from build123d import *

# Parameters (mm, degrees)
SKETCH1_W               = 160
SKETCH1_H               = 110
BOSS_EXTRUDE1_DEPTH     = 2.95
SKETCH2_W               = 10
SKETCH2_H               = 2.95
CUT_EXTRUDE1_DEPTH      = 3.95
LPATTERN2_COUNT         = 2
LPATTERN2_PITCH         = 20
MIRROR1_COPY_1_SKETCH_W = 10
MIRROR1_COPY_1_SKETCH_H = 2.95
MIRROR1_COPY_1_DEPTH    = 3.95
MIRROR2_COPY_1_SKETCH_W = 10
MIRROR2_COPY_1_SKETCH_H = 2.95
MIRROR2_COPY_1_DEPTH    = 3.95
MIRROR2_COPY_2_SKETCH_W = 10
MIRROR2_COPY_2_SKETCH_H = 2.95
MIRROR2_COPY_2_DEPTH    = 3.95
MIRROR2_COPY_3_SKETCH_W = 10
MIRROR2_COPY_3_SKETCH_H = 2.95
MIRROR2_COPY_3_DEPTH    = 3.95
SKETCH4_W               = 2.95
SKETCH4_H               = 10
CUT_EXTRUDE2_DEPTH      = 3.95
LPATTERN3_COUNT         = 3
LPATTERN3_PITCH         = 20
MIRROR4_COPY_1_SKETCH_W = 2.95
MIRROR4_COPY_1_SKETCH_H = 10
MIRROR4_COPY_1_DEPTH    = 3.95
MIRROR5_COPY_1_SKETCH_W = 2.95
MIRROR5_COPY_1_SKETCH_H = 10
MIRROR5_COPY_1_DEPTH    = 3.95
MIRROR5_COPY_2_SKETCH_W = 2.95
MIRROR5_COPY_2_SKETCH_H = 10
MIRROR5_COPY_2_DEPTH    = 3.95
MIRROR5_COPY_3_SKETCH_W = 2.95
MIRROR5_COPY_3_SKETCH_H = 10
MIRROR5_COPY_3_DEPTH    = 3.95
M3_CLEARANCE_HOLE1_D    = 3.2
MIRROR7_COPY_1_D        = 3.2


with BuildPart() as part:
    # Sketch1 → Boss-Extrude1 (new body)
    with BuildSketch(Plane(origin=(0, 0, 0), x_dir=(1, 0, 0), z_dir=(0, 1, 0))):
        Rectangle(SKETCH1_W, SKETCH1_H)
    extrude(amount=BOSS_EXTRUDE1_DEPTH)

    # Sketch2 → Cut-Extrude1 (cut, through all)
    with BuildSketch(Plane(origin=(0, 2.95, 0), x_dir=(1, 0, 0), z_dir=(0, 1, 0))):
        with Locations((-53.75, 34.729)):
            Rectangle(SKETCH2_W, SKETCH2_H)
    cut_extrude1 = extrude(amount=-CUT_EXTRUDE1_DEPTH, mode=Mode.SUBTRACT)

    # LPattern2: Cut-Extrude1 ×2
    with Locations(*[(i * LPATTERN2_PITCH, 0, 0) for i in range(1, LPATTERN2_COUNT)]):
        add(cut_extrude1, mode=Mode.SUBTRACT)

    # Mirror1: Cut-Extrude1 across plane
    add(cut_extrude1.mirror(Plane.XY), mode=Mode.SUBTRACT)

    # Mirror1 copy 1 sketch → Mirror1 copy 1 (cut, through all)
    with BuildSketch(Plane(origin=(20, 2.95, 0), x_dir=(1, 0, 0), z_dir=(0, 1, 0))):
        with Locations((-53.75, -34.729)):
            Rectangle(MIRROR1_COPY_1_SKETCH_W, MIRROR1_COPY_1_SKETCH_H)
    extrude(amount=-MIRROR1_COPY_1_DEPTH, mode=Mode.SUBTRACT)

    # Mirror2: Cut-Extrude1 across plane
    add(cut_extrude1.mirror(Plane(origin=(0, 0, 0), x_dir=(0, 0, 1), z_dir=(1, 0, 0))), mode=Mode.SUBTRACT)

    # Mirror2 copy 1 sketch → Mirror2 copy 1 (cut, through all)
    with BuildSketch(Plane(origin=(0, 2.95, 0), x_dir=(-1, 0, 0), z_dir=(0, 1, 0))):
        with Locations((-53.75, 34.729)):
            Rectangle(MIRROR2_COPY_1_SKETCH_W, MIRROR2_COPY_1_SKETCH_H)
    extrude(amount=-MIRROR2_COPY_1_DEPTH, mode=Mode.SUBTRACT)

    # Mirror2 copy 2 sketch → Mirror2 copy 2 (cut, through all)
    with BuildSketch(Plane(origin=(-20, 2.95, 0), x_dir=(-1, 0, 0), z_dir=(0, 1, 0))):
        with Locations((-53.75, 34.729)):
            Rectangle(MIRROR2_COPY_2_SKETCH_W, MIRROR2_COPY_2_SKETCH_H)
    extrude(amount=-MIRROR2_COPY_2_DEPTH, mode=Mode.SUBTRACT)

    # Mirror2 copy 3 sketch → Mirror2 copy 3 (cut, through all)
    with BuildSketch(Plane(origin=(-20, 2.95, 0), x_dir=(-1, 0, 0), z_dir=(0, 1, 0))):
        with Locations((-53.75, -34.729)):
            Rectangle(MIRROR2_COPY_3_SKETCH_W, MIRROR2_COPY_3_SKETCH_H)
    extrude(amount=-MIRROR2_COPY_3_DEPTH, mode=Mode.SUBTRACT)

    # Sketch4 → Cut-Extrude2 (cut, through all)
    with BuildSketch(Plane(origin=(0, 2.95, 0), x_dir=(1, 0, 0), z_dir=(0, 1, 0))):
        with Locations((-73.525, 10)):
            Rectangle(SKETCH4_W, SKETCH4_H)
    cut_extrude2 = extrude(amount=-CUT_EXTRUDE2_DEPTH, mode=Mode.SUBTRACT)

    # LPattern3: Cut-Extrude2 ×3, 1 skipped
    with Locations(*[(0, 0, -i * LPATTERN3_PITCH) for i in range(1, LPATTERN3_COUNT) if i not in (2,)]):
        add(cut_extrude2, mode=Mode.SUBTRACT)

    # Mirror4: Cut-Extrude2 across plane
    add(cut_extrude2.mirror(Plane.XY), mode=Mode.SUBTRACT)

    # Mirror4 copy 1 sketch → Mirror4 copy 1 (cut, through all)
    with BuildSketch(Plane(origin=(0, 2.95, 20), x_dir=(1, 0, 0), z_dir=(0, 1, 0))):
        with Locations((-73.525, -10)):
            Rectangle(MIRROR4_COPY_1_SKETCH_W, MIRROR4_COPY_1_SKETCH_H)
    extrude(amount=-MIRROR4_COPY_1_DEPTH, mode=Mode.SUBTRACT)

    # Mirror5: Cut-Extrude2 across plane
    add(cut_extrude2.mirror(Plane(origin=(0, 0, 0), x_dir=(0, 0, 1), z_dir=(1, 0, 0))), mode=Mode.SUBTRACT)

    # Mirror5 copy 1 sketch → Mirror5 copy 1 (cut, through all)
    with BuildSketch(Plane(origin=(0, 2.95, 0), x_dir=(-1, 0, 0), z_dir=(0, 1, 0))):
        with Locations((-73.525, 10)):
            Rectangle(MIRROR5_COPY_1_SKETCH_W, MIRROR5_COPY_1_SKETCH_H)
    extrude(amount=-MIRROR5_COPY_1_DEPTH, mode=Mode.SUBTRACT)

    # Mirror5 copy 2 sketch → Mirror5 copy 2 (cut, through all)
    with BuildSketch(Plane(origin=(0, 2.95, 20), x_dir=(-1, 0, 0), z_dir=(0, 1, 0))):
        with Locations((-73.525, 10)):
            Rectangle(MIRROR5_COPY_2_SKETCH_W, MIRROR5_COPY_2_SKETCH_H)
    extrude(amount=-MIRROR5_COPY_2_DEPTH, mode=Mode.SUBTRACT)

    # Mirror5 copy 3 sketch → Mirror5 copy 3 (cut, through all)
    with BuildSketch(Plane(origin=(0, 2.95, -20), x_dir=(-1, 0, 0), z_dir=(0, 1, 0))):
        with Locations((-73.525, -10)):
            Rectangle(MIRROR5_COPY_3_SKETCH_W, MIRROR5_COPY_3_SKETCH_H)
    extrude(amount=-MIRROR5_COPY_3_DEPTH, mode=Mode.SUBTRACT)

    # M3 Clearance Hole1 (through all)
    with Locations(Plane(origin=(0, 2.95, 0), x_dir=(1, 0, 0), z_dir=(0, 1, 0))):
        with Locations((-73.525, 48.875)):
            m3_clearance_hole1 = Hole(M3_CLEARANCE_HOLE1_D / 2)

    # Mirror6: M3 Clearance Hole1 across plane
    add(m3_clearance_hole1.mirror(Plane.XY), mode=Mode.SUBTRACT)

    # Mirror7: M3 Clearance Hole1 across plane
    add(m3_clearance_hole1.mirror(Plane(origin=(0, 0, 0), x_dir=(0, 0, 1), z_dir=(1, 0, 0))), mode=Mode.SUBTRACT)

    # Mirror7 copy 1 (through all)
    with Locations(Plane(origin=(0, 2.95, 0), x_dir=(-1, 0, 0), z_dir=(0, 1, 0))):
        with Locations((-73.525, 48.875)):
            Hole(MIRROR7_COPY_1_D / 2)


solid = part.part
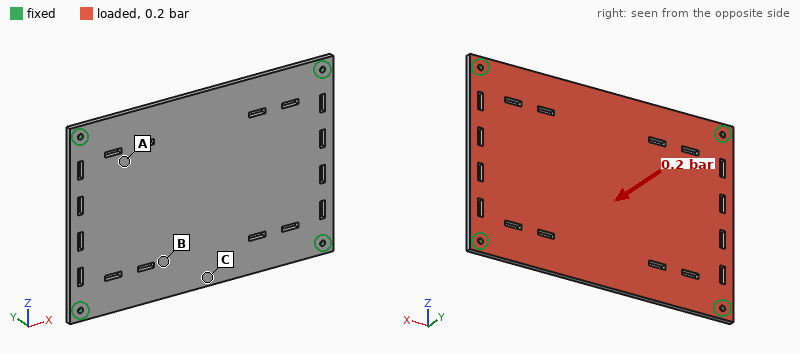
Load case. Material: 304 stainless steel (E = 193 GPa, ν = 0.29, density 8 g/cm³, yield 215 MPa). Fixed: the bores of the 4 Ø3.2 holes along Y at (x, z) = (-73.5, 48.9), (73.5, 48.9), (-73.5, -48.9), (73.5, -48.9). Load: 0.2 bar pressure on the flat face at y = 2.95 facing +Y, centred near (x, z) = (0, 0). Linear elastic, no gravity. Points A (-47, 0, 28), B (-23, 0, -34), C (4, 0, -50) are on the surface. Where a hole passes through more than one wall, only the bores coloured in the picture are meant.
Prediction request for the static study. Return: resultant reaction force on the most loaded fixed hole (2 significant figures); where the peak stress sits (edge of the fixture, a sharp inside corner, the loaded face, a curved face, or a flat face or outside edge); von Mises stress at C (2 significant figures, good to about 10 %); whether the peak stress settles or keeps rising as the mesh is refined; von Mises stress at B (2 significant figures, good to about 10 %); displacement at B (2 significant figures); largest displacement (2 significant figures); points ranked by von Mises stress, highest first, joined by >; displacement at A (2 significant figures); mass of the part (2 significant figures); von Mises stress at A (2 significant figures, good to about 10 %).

85 N
edge of the fixture
18 MPa
keeps rising
12 MPa
0.088 mm
0.11 mm
C > B > A
0.054 mm
400 g
6.0 MPa
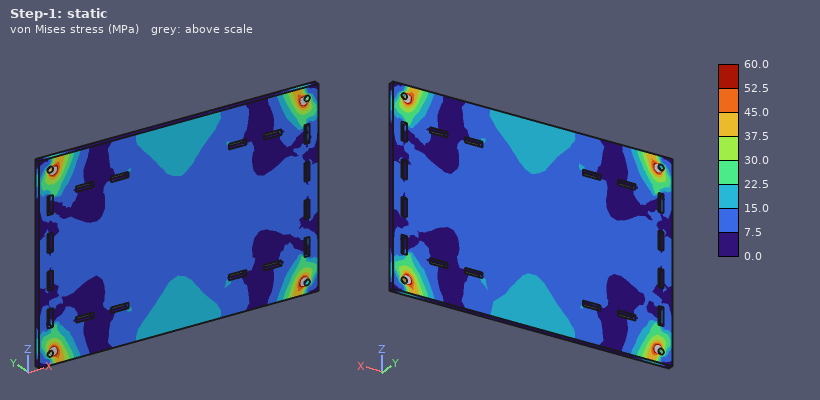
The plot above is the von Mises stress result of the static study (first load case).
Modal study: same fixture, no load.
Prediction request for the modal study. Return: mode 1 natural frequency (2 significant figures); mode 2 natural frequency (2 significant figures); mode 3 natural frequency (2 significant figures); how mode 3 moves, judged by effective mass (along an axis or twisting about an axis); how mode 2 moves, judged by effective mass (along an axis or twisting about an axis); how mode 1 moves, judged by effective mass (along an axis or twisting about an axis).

510 Hz
880 Hz
1300 Hz
twisting about Z
twisting about X
along Y
